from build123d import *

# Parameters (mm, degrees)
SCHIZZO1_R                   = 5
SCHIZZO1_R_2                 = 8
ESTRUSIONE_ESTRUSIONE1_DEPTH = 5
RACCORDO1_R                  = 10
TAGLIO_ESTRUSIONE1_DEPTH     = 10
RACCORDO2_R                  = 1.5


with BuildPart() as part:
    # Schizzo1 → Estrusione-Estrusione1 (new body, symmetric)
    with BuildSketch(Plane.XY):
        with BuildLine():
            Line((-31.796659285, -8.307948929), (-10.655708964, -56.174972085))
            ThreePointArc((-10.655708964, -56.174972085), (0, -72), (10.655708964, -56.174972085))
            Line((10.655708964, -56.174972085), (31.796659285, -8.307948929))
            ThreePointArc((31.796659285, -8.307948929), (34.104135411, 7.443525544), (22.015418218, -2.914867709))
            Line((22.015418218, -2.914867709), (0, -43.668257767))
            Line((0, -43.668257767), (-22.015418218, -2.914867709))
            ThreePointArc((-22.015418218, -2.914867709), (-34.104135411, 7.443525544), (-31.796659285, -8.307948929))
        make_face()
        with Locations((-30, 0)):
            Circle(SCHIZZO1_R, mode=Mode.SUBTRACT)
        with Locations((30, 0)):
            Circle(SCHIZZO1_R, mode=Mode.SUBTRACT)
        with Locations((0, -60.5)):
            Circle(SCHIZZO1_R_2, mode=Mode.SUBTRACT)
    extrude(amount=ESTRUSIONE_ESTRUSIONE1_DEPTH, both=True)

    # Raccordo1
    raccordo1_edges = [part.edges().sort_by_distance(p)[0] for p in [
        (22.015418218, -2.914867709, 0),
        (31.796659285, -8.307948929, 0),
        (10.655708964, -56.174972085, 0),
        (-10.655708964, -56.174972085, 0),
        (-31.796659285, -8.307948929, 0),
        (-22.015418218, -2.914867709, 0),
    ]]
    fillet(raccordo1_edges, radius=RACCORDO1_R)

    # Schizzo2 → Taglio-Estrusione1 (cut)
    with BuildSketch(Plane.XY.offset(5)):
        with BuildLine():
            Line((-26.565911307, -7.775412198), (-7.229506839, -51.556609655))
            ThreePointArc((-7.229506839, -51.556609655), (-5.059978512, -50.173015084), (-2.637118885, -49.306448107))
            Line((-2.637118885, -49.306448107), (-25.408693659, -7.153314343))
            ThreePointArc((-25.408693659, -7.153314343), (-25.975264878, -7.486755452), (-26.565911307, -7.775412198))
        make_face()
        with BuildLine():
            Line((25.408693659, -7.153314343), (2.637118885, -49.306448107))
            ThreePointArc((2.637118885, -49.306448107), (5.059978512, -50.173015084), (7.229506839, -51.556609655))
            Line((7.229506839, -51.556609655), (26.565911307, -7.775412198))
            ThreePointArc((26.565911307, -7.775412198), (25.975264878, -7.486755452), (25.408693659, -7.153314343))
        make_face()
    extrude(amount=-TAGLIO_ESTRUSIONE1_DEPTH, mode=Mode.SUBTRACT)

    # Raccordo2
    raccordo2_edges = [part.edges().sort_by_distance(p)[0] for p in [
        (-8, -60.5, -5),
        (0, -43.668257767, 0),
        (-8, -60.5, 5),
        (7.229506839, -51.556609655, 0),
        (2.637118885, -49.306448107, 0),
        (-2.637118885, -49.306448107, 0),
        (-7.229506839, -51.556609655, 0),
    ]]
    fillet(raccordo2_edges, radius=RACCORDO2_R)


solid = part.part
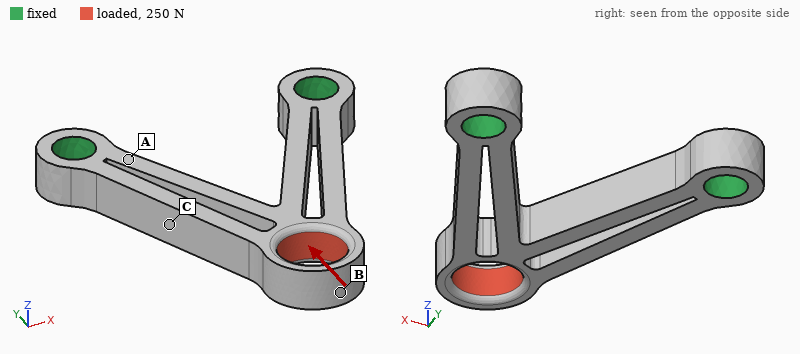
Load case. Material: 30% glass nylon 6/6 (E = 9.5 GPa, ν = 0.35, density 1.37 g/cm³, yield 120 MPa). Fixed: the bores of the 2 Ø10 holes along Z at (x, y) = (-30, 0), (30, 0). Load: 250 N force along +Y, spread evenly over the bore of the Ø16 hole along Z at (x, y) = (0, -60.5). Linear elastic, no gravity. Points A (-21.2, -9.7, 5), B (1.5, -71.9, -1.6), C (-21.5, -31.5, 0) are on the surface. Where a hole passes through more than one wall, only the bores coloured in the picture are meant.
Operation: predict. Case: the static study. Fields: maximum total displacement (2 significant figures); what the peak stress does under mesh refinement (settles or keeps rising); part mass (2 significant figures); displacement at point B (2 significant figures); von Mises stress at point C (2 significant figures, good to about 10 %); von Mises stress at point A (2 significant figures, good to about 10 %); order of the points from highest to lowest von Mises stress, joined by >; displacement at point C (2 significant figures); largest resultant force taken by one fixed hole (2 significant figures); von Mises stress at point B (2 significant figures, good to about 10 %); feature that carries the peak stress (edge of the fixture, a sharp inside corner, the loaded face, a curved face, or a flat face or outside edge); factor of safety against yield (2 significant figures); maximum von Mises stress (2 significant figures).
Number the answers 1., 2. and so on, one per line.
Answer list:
1. 20 µm
2. settles
3. 20 g
4. 19 µm
5. 2.0 MPa
6. 1.0 MPa
7. B > C > A
8. 6.1 µm
9. 140 N
10. 3.2 MPa
11. the loaded face
12. 19
13. 6.3 MPa
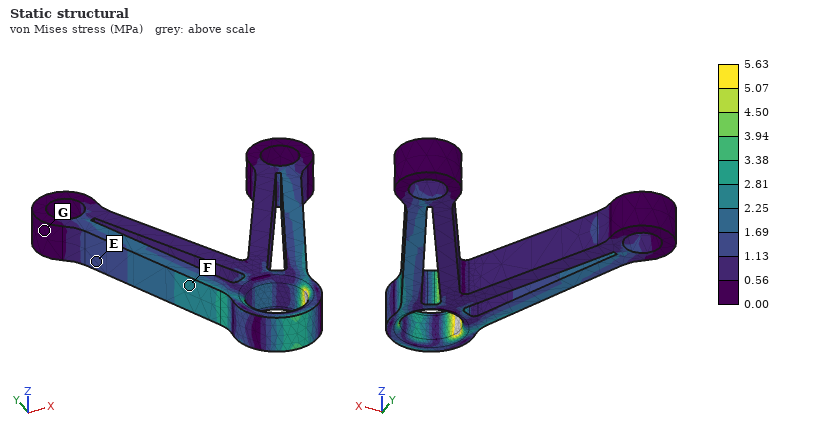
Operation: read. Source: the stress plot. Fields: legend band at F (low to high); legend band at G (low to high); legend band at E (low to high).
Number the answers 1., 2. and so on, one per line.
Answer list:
1. 2.25 to 2.81 MPa
2. 0.00 to 0.56 MPa
3. 1.13 to 1.69 MPa
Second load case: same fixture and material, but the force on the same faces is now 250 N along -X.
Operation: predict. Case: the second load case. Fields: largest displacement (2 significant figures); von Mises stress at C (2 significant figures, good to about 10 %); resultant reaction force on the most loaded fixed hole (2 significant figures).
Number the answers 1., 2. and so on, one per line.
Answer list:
1. 90 µm
2. 3.8 MPa
3. 280 N
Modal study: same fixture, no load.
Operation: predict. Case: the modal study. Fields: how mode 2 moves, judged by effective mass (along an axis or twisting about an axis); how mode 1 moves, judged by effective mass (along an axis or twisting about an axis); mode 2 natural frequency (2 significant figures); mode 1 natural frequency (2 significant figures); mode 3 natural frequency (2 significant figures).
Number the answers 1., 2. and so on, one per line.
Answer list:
1. along X
2. along Z
3. 3400 Hz
4. 1000 Hz
5. 3600 Hz
